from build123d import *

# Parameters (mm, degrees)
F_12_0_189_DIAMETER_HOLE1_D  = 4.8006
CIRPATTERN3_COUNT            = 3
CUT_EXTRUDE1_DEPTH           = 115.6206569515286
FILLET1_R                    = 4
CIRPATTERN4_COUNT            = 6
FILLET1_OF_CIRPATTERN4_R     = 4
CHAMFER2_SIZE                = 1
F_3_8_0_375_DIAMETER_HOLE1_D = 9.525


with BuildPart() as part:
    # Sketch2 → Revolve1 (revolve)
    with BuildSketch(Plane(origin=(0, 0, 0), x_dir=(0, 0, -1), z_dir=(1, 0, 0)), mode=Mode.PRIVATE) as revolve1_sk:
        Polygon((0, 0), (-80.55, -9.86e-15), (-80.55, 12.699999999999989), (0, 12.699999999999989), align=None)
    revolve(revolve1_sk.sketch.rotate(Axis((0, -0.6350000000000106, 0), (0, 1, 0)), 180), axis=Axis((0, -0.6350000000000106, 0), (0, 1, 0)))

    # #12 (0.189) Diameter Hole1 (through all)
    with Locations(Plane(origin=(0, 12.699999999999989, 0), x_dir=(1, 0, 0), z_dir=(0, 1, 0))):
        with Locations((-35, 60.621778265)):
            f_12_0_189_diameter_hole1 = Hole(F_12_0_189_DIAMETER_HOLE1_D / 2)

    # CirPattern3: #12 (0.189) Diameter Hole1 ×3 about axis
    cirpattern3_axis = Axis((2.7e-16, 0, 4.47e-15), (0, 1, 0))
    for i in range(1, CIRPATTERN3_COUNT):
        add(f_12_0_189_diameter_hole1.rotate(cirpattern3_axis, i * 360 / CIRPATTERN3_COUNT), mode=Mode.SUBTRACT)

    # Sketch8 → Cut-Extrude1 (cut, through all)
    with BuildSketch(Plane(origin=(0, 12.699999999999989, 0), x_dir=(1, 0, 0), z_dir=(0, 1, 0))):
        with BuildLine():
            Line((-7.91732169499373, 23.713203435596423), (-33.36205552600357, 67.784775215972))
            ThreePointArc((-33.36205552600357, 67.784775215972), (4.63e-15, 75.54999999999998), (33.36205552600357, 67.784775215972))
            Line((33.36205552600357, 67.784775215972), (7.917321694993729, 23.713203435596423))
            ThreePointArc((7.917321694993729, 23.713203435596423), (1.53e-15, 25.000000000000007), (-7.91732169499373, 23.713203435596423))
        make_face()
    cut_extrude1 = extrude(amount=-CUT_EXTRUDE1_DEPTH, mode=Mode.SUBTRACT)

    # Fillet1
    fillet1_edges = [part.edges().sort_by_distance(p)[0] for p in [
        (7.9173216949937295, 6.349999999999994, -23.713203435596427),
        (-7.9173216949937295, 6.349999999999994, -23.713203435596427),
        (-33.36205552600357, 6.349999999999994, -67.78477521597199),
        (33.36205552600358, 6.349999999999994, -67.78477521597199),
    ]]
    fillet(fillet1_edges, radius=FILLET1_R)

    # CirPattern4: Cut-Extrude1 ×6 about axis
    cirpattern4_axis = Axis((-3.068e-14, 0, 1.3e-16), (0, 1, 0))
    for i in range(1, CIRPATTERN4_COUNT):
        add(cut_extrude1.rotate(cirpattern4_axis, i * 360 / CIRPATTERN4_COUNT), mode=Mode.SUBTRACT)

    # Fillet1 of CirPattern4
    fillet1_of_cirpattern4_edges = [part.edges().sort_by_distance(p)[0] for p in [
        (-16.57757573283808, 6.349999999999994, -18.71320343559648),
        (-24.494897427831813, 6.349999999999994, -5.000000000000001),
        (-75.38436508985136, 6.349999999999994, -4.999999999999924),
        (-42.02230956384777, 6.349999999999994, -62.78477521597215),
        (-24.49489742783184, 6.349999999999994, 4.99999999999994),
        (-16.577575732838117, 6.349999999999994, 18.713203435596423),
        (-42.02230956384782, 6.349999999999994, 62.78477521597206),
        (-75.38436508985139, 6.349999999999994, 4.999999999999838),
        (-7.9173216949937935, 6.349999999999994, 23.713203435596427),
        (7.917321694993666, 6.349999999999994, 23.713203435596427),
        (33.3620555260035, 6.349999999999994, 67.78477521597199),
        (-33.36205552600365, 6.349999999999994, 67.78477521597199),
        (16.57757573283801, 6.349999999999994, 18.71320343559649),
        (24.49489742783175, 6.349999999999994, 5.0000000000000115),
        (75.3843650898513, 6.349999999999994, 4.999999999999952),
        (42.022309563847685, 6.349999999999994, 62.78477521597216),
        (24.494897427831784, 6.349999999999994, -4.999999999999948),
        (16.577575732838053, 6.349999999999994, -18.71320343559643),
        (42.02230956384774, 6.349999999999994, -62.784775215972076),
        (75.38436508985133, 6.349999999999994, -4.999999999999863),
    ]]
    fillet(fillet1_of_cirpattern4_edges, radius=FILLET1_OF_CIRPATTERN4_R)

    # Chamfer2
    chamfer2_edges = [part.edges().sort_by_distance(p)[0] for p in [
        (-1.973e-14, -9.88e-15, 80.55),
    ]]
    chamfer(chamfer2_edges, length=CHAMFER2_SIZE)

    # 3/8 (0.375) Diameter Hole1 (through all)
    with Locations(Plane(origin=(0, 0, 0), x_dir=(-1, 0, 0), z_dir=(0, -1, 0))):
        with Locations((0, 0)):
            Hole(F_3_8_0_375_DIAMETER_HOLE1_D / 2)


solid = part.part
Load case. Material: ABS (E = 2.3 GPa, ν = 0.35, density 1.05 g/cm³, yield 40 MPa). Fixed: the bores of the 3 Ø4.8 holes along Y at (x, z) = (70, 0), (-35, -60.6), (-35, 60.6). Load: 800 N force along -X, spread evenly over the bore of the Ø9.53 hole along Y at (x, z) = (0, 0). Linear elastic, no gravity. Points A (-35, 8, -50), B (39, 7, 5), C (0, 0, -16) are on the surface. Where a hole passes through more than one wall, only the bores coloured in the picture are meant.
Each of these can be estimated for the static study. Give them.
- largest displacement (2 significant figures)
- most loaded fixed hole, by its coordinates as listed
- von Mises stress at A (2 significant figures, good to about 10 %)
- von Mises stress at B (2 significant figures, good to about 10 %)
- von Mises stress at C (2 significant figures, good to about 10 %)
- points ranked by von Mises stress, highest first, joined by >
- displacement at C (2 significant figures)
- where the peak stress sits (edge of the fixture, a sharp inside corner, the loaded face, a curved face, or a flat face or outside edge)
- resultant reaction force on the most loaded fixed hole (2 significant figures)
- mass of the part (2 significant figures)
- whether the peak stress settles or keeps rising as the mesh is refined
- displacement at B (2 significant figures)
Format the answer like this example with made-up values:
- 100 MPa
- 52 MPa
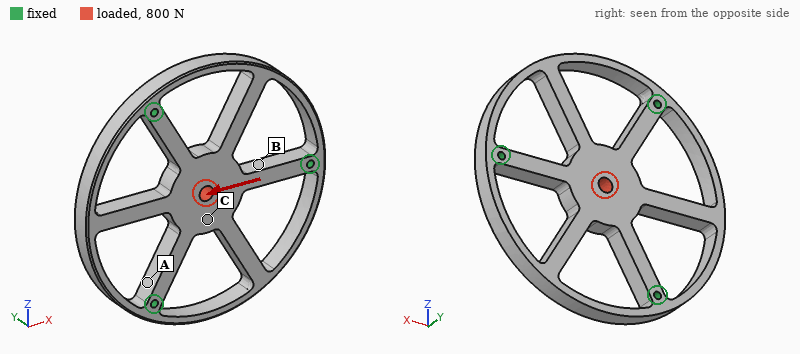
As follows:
- 0.11 mm
- (70, 0)
- 3.2 MPa
- 3.8 MPa
- 0.72 MPa
- B > A > C
- 0.089 mm
- edge of the fixture
- 480 N
- 98 g
- keeps rising
- 0.050 mm
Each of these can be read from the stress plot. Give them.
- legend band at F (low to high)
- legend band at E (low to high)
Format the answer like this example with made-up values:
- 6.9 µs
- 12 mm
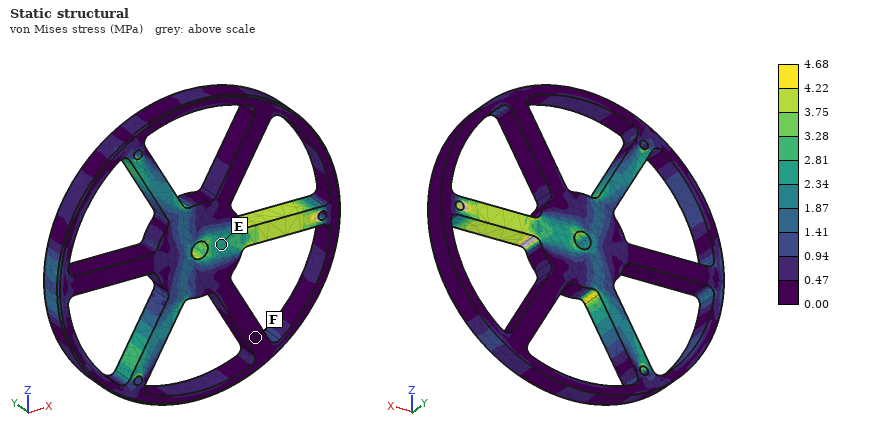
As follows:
- 0.00 to 0.47 MPa
- 2.34 to 2.81 MPa
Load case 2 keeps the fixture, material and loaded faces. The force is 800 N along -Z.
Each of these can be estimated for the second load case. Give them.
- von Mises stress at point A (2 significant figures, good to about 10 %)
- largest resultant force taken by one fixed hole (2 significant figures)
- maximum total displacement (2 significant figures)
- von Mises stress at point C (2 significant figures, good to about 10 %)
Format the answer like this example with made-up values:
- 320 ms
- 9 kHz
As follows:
- 2.5 MPa
- 420 N
- 0.11 mm
- 1.4 MPa
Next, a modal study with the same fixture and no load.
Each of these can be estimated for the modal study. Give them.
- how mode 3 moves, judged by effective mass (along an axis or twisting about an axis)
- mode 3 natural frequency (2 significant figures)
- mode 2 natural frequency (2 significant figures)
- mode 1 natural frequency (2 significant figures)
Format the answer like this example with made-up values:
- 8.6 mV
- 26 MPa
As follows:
- along Y
- 590 Hz
- 550 Hz
- 550 Hz
